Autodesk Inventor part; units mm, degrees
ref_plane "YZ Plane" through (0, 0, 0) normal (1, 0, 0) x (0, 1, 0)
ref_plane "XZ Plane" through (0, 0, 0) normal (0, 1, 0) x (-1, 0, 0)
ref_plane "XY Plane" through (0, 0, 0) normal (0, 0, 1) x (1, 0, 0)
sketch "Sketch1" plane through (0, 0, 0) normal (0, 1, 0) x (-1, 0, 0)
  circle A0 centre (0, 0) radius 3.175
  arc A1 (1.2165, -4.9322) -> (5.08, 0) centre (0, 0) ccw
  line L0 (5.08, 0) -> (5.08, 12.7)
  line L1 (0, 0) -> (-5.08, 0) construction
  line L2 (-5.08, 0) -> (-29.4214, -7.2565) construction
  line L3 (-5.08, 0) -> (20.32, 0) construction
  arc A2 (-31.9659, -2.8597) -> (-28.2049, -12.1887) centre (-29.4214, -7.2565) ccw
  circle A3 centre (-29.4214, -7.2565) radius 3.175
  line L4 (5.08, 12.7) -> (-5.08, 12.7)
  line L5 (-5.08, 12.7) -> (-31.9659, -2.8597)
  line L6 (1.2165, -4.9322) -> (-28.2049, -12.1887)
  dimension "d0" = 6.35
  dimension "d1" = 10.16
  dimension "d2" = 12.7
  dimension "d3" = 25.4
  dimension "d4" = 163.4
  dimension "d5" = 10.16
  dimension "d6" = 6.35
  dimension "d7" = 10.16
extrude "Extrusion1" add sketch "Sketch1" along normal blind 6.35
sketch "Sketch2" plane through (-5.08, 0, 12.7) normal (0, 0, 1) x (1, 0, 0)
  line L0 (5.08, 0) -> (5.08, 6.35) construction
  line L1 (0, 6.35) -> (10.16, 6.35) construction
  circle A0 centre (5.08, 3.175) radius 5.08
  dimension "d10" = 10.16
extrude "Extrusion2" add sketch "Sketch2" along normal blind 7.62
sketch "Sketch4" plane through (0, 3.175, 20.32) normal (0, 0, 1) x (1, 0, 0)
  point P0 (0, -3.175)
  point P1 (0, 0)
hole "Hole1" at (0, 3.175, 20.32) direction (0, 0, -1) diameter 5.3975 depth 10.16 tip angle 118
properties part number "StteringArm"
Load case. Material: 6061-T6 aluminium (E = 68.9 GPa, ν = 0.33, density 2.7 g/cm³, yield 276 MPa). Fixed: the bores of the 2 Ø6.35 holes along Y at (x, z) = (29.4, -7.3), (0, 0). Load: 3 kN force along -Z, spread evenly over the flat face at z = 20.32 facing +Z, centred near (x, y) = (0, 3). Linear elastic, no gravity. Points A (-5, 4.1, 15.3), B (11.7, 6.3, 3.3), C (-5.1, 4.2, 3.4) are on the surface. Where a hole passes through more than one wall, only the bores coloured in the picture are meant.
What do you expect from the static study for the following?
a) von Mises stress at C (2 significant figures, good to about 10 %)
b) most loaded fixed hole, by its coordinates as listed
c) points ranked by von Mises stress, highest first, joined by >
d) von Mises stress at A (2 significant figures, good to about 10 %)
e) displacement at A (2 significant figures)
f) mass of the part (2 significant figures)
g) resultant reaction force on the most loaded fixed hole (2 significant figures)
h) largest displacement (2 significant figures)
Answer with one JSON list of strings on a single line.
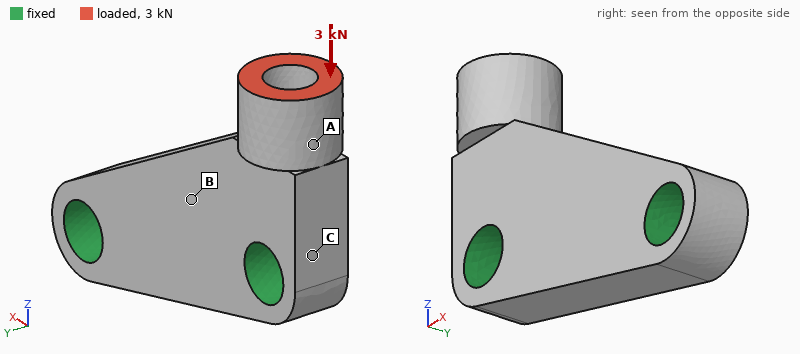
["44 MPa", "(0, 0)", "A > C > B", "65 MPa", "14 µm", "10 g", "2.9 kN", "19 µm"]
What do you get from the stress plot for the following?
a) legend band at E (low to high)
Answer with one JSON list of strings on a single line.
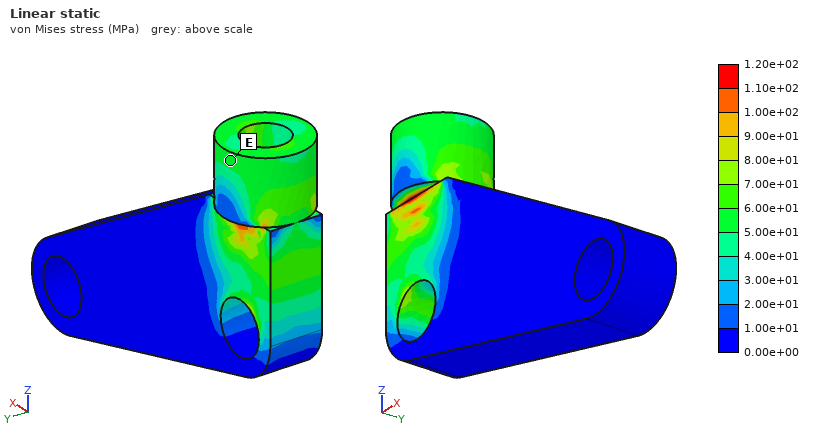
["5.00e+01 to 6.00e+01 MPa"]
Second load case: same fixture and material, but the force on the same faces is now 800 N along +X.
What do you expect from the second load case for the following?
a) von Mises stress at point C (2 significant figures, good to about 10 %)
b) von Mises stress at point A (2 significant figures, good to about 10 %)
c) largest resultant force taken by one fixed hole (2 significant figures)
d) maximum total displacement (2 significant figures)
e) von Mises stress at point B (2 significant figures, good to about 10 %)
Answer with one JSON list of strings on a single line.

["46 MPa", "43 MPa", "630 N", "39 µm", "14 MPa"]
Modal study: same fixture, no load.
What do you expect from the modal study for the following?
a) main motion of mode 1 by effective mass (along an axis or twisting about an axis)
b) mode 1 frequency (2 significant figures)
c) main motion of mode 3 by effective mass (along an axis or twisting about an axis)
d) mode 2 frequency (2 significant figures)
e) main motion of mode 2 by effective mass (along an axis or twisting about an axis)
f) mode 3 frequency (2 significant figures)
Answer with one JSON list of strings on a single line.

["along Y", "16 kHz", "along Y", "28 kHz", "along X", "29 kHz"]
